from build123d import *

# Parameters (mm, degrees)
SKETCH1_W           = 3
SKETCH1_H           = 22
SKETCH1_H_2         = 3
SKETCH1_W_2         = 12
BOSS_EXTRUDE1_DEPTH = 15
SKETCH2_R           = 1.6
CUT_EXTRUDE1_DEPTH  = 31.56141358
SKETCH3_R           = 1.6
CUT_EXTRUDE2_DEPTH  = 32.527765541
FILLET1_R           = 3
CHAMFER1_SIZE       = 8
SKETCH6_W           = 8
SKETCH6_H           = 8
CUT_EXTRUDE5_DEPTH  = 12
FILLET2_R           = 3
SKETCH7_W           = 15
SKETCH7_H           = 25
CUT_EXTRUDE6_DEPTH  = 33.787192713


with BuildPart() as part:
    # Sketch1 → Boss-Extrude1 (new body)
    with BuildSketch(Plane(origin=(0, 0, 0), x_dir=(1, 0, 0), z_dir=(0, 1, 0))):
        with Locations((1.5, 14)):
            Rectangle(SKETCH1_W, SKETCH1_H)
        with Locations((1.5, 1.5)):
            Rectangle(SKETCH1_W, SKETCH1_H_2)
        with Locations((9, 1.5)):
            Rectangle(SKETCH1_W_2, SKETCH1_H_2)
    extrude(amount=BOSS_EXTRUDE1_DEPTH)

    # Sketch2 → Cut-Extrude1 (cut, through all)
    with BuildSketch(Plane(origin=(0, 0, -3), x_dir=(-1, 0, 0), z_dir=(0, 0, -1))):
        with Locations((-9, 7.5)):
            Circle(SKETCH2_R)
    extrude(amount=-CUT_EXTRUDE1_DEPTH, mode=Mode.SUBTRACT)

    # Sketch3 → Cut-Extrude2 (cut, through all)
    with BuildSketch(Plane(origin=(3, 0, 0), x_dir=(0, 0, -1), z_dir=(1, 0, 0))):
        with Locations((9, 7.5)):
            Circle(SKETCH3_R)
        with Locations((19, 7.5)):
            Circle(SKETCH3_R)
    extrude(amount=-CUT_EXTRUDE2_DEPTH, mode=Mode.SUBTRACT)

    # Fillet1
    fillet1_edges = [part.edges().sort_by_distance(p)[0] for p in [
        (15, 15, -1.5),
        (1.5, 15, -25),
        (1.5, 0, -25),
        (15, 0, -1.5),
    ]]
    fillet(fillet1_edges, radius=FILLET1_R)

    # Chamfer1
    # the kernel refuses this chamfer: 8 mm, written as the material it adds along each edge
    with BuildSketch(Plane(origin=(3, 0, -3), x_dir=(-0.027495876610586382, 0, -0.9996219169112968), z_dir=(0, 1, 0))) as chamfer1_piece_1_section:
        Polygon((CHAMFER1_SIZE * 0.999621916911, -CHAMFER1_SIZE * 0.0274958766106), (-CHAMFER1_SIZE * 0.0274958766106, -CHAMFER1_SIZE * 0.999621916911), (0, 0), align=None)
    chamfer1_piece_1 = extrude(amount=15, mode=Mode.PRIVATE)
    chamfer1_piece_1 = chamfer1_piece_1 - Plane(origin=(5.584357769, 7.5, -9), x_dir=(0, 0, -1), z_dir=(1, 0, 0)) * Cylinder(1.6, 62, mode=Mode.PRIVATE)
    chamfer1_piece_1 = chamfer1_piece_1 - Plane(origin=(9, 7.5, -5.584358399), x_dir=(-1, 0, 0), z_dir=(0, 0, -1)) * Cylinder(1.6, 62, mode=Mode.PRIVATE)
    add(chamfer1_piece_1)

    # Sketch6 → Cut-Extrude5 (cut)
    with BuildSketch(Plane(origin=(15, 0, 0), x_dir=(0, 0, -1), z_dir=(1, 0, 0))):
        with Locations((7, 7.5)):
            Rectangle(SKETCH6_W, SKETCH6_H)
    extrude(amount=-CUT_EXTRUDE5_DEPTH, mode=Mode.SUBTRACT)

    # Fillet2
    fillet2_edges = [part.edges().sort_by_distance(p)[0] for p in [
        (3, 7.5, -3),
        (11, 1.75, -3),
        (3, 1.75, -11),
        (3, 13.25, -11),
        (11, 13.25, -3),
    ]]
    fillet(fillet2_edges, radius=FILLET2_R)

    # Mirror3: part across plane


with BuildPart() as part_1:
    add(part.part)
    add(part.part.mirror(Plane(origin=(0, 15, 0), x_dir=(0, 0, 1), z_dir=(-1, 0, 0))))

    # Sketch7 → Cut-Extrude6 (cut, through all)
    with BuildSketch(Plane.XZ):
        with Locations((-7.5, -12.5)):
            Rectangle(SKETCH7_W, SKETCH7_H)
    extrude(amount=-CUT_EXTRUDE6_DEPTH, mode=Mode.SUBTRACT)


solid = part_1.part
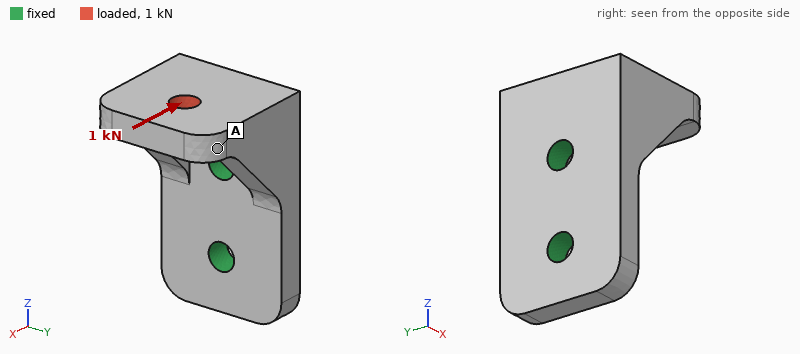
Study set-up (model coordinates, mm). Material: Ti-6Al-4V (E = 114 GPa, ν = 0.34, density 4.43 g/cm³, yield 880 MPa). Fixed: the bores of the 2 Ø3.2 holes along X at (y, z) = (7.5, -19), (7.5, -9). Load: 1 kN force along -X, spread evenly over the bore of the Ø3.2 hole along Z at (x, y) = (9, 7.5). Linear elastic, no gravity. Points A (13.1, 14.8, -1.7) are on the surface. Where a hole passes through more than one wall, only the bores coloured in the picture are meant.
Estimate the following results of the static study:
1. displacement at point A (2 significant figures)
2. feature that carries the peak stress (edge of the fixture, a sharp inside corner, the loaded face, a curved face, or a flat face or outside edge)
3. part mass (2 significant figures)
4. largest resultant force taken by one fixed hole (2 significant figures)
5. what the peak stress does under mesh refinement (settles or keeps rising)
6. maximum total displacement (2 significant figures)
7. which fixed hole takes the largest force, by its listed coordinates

47 µm
edge of the fixture
8.0 g
1.3 kN
keeps rising
57 µm
(7.5, -9)
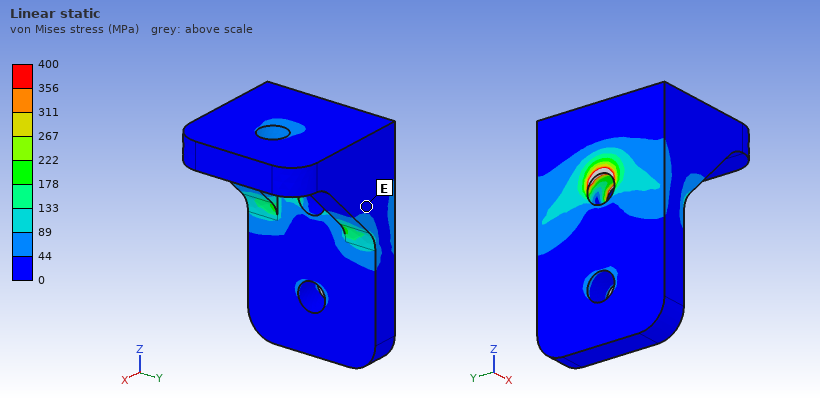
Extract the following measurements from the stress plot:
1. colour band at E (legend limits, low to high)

0 to 44 MPa
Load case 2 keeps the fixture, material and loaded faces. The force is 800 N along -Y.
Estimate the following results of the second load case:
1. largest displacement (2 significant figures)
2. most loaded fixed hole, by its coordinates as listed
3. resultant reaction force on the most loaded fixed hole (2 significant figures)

57 µm
(7.5, -9)
1.2 kN
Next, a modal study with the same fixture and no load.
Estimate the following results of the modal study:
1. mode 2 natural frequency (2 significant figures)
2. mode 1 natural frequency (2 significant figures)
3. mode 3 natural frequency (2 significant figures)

12 kHz
12 kHz
29 kHz
